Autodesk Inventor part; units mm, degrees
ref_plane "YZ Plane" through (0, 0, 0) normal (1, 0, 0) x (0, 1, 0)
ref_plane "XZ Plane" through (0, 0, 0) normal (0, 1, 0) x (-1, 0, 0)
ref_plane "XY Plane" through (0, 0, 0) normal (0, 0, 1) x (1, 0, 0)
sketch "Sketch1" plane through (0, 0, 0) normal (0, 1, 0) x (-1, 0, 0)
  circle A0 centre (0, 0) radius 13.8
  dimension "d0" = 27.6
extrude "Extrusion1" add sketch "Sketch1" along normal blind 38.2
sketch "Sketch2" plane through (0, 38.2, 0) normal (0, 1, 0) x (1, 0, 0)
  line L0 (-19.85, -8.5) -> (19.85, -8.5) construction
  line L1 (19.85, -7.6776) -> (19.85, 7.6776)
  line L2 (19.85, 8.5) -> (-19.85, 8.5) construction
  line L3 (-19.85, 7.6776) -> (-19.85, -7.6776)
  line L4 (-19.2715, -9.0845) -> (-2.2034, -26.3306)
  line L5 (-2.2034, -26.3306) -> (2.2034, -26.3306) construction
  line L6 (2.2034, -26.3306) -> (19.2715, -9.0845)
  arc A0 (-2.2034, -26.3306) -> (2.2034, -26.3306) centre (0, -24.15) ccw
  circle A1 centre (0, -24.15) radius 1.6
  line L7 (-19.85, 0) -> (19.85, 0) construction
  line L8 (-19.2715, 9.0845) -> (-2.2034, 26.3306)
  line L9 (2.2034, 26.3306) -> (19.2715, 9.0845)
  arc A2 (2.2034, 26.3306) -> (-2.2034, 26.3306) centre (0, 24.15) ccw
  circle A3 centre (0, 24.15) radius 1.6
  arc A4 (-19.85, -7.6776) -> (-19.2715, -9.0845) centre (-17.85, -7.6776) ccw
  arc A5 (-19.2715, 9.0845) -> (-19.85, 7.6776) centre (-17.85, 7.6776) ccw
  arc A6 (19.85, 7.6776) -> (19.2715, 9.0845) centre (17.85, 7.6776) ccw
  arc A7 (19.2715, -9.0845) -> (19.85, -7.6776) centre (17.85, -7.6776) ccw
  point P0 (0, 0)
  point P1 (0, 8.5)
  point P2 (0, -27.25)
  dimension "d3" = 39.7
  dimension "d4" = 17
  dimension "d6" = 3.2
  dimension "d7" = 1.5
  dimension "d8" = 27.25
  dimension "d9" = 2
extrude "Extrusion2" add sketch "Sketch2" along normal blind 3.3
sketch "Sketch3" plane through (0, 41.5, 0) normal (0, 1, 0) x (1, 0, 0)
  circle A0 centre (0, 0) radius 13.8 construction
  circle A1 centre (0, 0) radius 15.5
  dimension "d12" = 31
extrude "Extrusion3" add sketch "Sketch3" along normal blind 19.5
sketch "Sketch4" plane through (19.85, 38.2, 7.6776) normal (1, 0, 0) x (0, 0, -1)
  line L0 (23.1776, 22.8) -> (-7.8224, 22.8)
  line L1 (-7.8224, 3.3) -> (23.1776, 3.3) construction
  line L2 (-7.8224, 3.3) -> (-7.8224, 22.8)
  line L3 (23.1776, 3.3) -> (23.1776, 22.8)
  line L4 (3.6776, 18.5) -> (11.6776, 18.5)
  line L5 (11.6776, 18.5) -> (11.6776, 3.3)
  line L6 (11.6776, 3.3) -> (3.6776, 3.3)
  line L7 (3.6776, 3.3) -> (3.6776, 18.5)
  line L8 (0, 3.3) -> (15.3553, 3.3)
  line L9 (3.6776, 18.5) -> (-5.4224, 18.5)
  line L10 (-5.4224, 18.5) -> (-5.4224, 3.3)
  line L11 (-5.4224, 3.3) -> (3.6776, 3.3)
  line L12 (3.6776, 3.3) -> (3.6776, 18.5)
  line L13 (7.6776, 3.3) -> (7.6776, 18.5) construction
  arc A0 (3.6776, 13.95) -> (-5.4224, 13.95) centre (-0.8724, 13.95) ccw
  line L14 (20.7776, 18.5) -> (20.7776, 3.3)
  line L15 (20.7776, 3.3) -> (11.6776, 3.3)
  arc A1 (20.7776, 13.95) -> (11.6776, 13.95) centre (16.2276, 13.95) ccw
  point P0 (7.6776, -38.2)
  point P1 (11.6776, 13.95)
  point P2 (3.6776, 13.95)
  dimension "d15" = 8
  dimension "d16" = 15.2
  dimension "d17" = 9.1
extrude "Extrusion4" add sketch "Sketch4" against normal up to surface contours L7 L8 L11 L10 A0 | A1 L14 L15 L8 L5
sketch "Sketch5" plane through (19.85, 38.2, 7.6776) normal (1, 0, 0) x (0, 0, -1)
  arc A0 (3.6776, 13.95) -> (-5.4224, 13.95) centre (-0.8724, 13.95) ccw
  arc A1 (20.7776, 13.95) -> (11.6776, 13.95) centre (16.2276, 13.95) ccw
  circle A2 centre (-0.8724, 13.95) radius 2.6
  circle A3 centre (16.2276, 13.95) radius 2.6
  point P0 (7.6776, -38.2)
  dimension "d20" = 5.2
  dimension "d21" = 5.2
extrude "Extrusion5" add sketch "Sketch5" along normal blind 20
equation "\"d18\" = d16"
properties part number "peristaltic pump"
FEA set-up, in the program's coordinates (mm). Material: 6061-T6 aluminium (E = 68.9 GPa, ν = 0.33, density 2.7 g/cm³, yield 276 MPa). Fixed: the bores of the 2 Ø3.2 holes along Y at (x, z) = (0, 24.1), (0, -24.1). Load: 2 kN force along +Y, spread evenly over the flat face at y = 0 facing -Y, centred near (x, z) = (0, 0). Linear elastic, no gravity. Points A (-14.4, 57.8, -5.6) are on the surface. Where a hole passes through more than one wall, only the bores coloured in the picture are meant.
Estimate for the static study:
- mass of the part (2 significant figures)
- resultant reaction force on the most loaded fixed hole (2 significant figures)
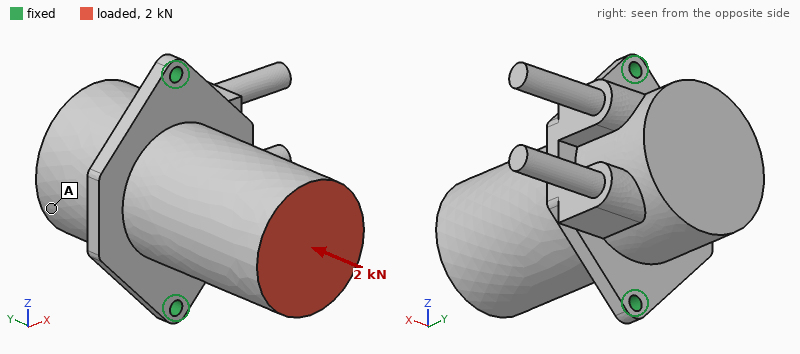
120 g
1.0 kN
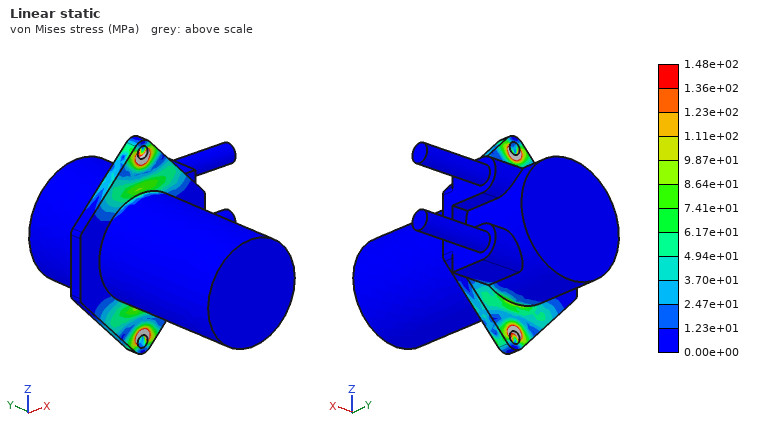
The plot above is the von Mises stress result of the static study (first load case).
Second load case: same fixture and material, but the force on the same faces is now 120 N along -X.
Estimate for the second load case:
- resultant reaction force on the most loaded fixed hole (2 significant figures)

60 N
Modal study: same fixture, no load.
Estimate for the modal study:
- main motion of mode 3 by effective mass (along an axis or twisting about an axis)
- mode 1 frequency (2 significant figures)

along Y
720 Hz
